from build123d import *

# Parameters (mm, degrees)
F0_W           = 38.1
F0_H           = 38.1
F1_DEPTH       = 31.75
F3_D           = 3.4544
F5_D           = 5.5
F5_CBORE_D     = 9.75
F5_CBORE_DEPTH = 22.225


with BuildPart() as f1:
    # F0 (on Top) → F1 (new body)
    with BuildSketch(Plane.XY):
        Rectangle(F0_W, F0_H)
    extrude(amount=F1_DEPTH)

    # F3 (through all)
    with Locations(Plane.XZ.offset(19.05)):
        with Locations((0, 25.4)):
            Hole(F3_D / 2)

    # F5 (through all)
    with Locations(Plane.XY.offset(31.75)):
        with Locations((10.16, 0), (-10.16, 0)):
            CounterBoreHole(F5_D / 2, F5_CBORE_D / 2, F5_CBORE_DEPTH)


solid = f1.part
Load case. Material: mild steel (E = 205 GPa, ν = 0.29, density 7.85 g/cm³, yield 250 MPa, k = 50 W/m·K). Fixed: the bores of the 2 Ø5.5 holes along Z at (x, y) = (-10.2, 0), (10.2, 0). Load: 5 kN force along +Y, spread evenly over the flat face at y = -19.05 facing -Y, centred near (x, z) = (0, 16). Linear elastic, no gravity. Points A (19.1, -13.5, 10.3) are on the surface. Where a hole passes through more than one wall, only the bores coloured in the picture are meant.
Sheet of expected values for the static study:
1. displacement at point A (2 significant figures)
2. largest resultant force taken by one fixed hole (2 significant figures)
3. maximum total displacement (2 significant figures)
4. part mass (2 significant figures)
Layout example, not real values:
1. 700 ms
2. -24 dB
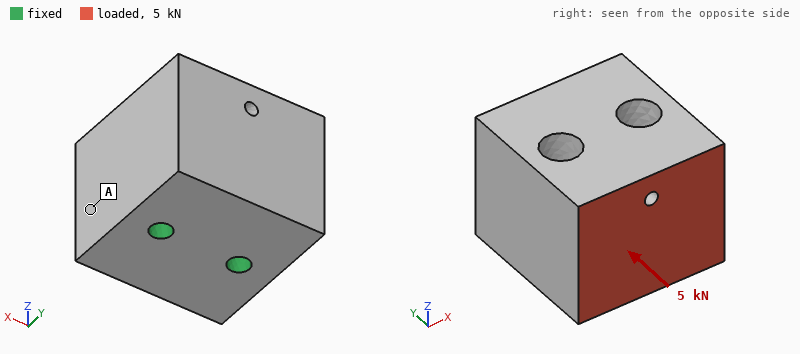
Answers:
1. 4.6 µm
2. 2.5 kN
3. 11 µm
4. 330 g
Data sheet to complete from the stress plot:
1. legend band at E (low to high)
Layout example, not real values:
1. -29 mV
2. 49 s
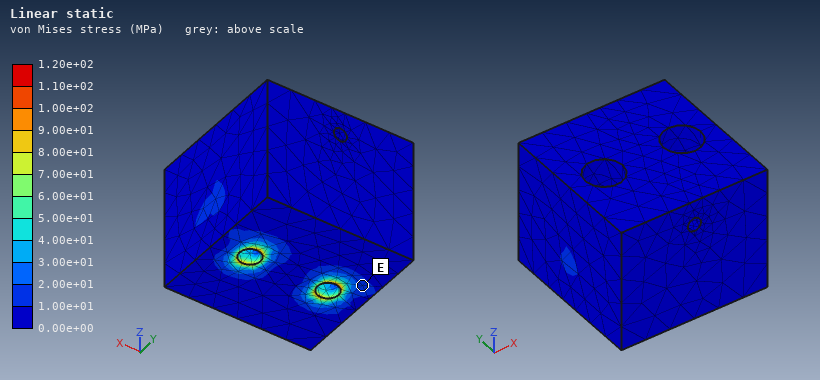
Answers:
1. 1.00e+01 to 2.00e+01 MPa
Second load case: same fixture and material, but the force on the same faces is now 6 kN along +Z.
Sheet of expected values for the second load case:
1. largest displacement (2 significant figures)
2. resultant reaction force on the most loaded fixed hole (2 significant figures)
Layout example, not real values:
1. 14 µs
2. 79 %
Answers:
1. 23 µm
2. 3.0 kN
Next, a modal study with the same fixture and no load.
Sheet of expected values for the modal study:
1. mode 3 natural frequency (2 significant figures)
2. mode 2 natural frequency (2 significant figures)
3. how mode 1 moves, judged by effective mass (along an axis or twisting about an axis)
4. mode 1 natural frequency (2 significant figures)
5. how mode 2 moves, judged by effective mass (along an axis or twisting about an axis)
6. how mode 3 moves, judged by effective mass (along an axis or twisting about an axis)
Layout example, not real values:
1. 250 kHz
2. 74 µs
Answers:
1. 16 kHz
2. 12 kHz
3. along Y
4. 6400 Hz
5. along X
6. twisting about Z
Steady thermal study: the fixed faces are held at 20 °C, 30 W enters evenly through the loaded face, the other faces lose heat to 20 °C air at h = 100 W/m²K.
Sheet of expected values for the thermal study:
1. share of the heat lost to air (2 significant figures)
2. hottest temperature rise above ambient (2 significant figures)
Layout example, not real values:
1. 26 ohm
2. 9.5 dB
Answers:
1. 18 %
2. 16 K
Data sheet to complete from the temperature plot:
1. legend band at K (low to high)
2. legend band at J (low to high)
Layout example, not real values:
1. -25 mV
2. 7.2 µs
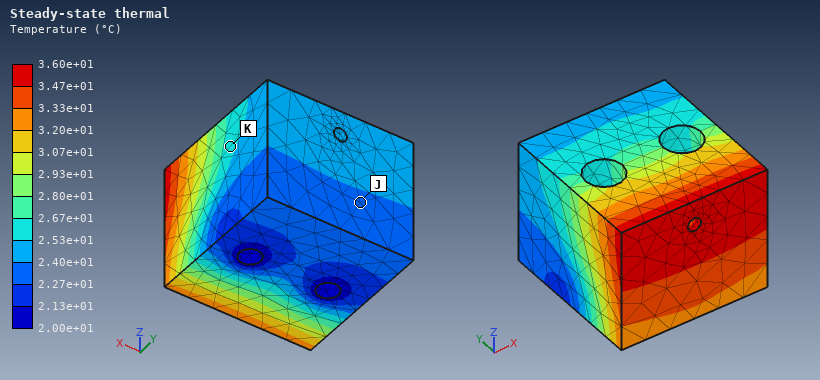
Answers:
1. 2.53e+01 to 2.67e+01 °C
2. 2.27e+01 to 2.40e+01 °C
